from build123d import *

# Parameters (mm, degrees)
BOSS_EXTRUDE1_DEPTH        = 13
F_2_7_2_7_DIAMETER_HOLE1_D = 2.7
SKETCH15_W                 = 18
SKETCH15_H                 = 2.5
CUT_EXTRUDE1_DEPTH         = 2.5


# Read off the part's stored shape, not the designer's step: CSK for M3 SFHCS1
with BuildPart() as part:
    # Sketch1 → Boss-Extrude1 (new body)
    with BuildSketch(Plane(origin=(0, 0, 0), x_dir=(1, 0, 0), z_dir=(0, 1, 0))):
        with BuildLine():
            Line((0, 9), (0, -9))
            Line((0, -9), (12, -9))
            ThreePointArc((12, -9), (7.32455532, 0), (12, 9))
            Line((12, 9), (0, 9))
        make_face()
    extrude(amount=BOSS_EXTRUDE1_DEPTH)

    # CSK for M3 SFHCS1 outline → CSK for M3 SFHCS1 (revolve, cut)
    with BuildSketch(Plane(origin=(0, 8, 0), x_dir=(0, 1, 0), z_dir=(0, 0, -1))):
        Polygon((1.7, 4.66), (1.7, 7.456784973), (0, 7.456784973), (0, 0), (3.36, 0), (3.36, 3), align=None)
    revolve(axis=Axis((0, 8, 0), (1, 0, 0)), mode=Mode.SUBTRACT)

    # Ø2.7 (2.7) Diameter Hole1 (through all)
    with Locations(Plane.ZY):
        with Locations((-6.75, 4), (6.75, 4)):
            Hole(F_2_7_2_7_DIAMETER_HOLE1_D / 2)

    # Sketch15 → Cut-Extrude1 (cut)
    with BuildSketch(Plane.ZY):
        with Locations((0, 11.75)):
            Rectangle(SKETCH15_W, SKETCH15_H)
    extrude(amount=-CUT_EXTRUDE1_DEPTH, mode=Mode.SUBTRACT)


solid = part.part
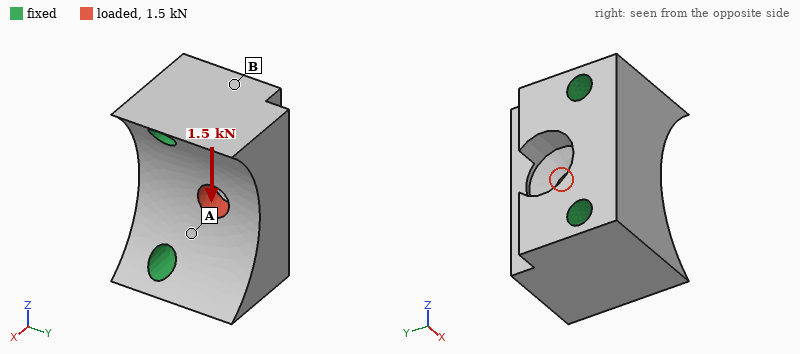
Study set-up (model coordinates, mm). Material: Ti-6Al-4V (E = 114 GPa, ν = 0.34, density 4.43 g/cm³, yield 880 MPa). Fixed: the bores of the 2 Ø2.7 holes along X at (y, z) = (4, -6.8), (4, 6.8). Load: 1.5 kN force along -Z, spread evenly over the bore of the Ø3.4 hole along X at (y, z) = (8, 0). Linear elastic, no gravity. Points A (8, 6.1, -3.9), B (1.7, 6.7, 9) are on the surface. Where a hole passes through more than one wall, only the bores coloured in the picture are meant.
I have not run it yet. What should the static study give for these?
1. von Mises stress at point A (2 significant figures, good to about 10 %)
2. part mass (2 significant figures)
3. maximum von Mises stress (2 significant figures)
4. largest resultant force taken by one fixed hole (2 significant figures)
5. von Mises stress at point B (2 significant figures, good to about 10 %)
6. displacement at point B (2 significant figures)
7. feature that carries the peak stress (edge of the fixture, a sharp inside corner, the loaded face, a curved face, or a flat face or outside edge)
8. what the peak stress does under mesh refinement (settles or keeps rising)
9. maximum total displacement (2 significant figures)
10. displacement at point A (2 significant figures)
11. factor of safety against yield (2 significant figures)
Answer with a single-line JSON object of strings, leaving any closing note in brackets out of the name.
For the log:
{"von Mises stress at point A": "36 MPa", "part mass": "7.3 g", "maximum von Mises stress": "92 MPa", "largest resultant force taken by one fixed hole": "820 N", "von Mises stress at point B": "13 MPa", "displacement at point B": "0.72 µm", "feature that carries the peak stress": "the loaded face", "what the peak stress does under mesh refinement": "settles", "maximum total displacement": "3.3 µm", "displacement at point A": "0.80 µm", "factor of safety against yield": "9.6"}
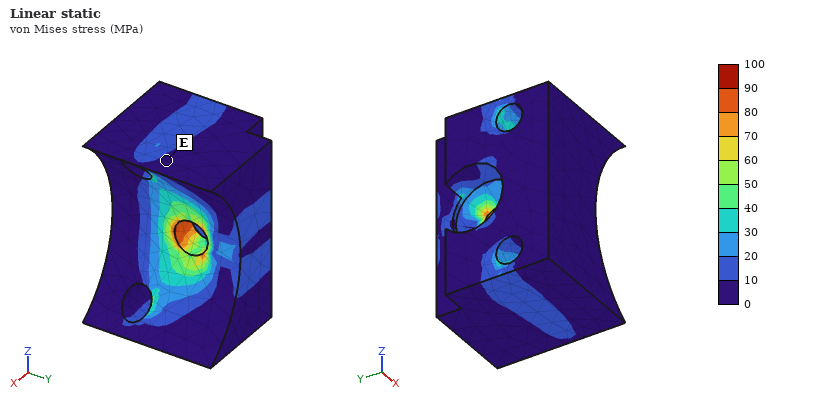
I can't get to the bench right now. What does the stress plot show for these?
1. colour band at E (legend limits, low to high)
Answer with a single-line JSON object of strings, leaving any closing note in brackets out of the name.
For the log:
{"colour band at E": "0 to 10 MPa"}
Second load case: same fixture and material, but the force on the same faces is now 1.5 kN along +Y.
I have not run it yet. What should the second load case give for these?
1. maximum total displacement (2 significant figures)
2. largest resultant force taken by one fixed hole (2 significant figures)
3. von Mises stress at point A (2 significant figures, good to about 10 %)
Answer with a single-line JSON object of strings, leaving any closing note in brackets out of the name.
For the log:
{"maximum total displacement": "3.7 µm", "largest resultant force taken by one fixed hole": "780 N", "von Mises stress at point A": "34 MPa"}
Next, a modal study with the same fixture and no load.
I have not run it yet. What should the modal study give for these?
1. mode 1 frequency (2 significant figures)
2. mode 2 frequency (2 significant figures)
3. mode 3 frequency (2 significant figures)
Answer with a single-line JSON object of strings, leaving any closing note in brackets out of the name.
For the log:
{"mode 1 frequency": "64 kHz", "mode 2 frequency": "65 kHz", "mode 3 frequency": "77 kHz"}
